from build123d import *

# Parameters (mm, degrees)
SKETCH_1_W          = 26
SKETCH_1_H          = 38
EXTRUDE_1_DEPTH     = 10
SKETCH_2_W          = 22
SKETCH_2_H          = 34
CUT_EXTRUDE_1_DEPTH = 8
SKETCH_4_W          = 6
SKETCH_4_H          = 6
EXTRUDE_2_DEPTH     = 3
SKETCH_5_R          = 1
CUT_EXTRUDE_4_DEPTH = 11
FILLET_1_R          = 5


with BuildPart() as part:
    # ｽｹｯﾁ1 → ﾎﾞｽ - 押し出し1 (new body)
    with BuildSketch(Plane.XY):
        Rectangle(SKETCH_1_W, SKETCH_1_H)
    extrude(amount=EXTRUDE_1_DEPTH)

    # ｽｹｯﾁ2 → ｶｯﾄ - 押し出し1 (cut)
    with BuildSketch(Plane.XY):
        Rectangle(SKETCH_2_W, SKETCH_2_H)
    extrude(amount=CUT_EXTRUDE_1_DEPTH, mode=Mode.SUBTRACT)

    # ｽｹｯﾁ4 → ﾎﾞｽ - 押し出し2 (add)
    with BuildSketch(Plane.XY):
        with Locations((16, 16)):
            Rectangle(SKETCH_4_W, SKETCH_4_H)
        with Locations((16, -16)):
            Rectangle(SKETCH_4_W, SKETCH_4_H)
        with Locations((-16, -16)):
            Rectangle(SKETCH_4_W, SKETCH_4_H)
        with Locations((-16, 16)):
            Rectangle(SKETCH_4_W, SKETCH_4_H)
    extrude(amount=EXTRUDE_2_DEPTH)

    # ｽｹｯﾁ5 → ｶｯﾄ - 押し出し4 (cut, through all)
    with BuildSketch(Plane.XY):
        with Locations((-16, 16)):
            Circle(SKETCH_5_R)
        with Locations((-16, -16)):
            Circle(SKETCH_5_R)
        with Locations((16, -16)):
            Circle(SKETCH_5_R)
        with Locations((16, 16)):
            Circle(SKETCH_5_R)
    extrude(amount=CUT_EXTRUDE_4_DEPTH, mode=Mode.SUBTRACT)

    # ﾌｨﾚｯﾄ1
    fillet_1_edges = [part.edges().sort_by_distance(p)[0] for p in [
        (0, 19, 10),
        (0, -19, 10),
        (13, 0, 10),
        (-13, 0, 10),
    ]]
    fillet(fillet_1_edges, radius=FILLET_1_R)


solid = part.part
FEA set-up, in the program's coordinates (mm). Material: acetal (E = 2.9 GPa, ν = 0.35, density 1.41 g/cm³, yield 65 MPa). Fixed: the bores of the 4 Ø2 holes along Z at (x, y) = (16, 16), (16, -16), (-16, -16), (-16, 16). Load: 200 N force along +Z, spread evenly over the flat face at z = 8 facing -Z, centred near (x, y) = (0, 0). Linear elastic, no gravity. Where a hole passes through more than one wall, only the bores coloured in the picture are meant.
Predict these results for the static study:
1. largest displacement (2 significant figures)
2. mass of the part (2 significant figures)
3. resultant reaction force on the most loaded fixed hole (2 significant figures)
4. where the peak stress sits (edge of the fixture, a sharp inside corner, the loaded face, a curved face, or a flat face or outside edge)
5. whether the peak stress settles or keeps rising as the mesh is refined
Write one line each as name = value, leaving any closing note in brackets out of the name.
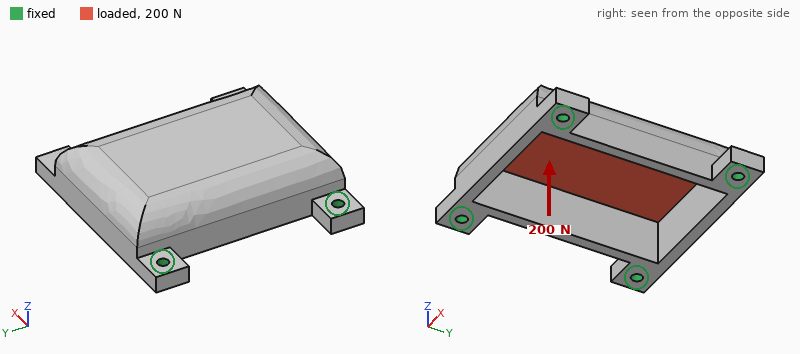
largest displacement = 0.25 mm
mass of the part = 5.1 g
resultant reaction force on the most loaded fixed hole = 61 N
where the peak stress sits = edge of the fixture
whether the peak stress settles or keeps rising as the mesh is refined = keeps rising
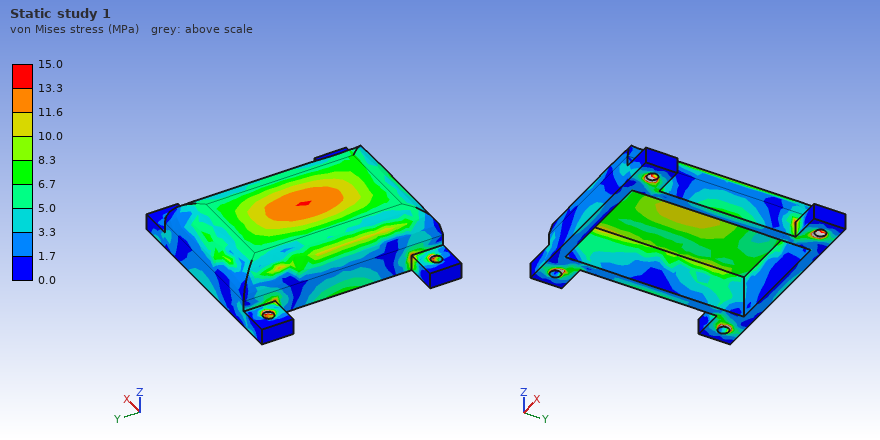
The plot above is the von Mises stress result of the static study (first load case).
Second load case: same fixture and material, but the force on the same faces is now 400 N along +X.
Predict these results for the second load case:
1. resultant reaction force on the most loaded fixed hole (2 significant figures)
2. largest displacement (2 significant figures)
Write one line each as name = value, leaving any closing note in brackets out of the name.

resultant reaction force on the most loaded fixed hole = 110 N
largest displacement = 0.14 mm
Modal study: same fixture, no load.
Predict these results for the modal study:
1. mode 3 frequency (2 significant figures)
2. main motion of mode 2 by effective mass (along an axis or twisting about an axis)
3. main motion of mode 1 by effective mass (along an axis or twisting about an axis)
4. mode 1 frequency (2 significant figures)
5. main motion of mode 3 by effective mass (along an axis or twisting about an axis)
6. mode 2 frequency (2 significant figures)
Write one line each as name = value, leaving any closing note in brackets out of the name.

mode 3 frequency = 5000 Hz
main motion of mode 2 by effective mass = along X
main motion of mode 1 by effective mass = along Z
mode 1 frequency = 3600 Hz
main motion of mode 3 by effective mass = along Y
mode 2 frequency = 4700 Hz
